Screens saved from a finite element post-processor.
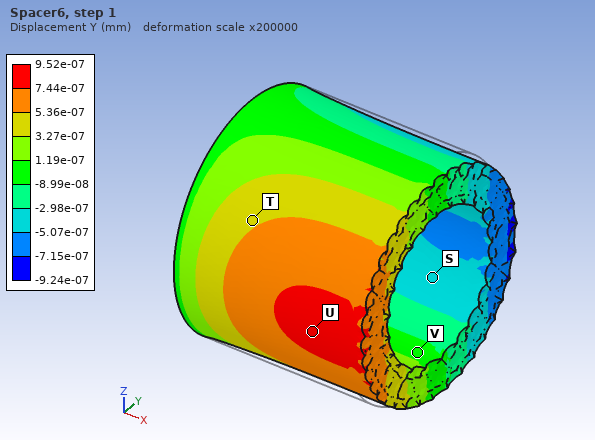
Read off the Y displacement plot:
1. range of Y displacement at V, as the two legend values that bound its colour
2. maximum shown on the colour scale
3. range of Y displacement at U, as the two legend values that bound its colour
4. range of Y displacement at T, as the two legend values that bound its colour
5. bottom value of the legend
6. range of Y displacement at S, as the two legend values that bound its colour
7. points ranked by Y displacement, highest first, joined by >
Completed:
-8.99e-08 to 1.19e-07 mm
9.52e-07 mm
7.44e-07 to 9.52e-07 mm
3.27e-07 to 5.36e-07 mm
-9.24e-07 mm
-5.07e-07 to -2.98e-07 mm
U > T > V > S
